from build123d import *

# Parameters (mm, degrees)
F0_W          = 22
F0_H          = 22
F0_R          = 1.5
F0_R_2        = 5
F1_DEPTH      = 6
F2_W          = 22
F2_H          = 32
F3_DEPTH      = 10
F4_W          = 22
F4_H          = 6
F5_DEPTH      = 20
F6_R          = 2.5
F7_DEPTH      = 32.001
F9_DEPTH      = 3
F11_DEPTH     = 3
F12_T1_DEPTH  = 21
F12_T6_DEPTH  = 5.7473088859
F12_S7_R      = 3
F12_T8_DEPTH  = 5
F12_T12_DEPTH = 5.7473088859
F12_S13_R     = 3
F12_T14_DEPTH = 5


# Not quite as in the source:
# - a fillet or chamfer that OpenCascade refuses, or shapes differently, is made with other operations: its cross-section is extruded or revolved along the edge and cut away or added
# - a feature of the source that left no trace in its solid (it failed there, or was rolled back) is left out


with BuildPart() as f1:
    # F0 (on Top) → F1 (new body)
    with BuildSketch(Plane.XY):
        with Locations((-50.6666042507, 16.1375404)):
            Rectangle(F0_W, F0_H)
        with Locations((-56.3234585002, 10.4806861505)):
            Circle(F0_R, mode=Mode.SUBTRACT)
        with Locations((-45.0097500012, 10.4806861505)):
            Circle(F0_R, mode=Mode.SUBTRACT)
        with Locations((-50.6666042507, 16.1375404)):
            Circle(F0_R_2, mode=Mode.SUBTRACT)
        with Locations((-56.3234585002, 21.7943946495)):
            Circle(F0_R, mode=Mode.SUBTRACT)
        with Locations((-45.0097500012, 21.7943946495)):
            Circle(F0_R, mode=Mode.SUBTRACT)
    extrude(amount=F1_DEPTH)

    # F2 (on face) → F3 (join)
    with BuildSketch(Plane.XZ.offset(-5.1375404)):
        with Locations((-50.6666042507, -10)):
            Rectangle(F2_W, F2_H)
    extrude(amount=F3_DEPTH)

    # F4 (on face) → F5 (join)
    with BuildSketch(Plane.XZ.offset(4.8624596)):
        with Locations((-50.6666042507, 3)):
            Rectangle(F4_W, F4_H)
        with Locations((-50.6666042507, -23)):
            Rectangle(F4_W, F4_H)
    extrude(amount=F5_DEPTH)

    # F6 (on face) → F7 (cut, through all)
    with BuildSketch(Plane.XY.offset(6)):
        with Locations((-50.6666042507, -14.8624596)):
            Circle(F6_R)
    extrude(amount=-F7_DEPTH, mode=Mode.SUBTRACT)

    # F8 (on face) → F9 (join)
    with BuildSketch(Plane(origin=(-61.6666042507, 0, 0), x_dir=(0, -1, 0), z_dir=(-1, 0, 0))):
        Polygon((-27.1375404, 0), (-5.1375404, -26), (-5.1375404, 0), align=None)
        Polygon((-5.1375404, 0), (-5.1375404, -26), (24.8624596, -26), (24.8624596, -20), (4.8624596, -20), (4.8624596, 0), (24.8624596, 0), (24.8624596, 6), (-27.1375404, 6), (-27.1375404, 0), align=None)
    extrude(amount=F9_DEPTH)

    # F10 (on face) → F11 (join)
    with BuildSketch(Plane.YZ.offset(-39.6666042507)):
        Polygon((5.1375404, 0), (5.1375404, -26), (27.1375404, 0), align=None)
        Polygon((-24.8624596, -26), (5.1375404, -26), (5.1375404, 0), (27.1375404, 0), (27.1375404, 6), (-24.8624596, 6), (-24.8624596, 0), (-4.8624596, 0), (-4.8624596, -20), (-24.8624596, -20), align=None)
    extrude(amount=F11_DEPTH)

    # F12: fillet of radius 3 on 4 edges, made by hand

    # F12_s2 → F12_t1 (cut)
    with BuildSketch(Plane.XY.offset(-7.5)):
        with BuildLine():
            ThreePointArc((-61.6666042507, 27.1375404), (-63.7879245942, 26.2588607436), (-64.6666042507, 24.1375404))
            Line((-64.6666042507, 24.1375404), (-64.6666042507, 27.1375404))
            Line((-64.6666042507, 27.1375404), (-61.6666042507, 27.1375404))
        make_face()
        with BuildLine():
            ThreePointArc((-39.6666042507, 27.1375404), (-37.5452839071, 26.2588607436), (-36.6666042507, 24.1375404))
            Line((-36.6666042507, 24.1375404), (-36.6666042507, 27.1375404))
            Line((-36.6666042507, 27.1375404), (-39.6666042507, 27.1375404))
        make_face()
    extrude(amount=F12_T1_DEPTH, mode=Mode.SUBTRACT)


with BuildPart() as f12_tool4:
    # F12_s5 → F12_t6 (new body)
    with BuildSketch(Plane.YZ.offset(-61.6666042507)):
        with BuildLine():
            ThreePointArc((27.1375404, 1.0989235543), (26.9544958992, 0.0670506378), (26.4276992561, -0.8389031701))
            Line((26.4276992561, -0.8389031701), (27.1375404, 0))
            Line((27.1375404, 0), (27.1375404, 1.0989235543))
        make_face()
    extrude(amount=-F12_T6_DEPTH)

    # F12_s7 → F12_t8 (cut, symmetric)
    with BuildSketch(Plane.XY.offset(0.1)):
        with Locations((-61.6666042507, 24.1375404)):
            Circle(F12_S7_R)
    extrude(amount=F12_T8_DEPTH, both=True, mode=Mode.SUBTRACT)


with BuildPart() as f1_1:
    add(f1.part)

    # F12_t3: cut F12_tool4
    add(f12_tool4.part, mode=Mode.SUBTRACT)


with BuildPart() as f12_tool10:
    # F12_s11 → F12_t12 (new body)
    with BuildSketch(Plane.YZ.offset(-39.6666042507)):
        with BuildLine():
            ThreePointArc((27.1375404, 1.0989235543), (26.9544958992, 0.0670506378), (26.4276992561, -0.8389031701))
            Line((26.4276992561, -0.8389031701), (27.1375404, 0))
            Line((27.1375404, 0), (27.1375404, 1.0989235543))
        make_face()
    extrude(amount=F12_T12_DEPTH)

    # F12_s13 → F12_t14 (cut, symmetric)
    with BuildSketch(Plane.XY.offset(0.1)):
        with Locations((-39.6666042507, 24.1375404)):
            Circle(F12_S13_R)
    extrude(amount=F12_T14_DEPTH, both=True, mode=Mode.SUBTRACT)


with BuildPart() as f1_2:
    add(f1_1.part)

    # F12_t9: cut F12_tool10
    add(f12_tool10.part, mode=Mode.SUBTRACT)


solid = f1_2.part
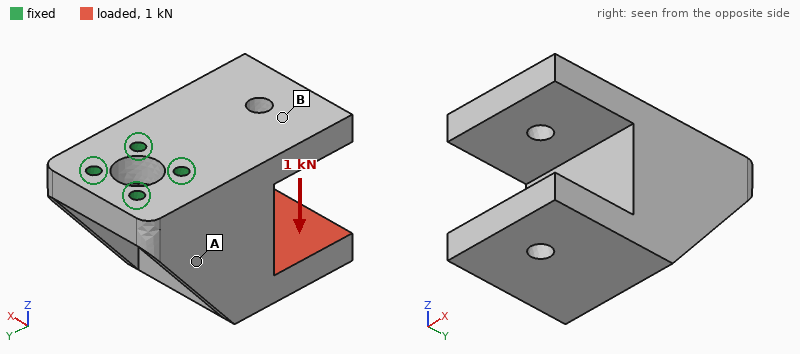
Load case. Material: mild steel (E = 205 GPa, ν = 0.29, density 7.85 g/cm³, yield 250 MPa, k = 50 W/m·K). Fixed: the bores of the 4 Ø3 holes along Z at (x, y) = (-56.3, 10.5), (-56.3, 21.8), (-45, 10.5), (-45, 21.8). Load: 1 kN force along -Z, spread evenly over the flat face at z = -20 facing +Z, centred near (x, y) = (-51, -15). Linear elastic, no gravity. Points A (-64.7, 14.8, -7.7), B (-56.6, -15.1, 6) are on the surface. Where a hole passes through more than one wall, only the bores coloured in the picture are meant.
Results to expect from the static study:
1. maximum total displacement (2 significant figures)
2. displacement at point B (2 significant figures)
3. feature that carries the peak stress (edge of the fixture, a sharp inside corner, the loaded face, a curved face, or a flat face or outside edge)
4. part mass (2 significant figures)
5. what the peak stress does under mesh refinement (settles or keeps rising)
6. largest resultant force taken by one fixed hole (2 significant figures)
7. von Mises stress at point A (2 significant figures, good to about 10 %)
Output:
44 µm
12 µm
edge of the fixture
160 g
keeps rising
1.1 kN
20 MPa
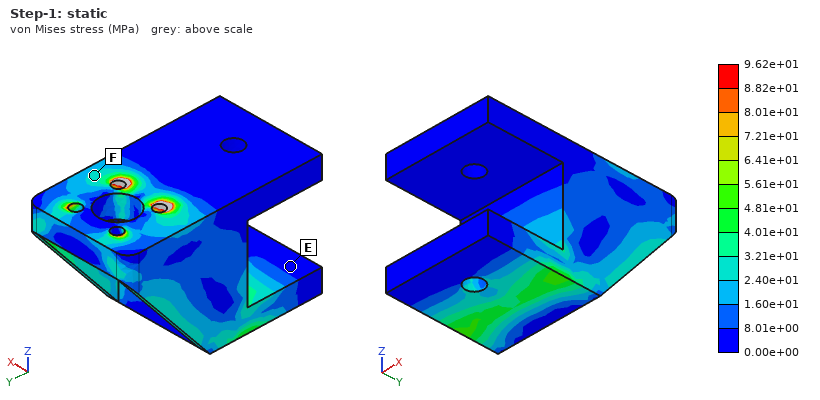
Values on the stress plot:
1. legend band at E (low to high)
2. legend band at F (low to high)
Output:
0.00e+00 to 8.01e+00 MPa
2.40e+01 to 3.21e+01 MPa
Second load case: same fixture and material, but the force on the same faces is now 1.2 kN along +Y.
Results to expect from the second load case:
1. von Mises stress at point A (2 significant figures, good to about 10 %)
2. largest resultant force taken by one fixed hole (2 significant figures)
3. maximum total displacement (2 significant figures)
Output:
25 MPa
790 N
20 µm
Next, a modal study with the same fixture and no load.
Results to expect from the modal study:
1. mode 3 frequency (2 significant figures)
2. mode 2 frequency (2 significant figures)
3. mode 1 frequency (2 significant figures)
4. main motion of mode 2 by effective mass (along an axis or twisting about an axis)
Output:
8100 Hz
5800 Hz
3800 Hz
along X
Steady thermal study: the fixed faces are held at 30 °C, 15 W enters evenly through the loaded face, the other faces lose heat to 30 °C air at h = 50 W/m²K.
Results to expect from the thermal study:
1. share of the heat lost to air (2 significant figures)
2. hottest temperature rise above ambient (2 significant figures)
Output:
34 %
45 K
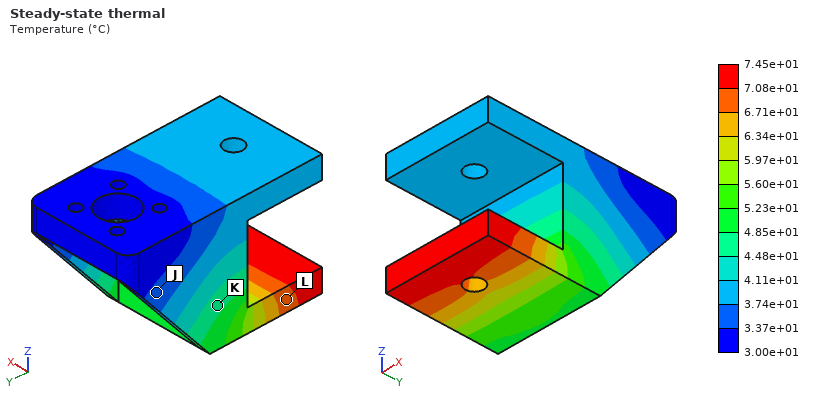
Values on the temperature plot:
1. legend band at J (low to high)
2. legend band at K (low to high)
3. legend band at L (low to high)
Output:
3.37e+01 to 3.74e+01 °C
4.48e+01 to 4.85e+01 °C
6.71e+01 to 7.08e+01 °C
